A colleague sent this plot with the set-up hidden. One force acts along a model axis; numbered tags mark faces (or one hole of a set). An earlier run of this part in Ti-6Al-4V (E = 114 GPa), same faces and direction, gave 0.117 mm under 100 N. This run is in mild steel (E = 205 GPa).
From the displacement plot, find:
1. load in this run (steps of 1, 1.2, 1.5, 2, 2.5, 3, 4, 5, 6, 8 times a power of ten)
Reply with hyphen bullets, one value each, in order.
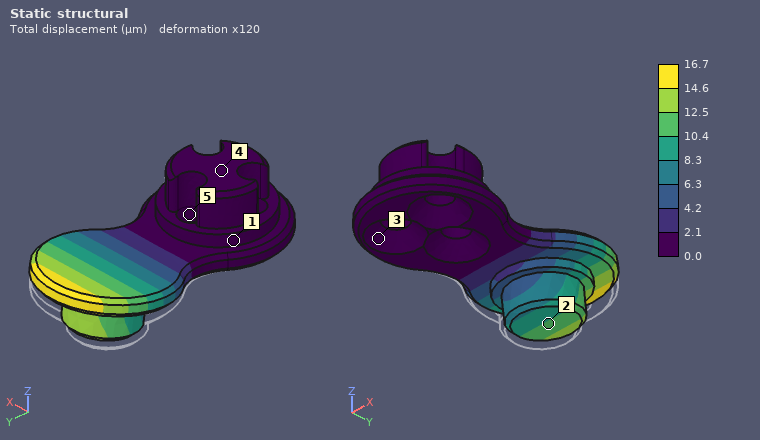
- 25 N
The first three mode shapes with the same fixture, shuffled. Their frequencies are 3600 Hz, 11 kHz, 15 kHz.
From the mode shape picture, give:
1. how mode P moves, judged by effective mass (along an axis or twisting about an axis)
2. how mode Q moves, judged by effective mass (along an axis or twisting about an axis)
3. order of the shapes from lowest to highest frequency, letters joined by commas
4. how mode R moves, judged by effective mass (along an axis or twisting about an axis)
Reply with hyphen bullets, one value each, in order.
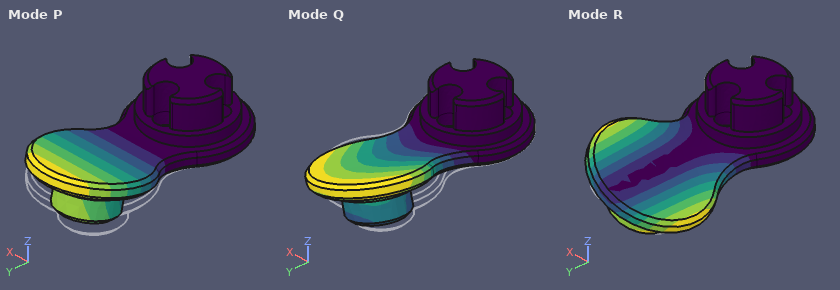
- along Z
- along X
- P, R, Q
- along X
